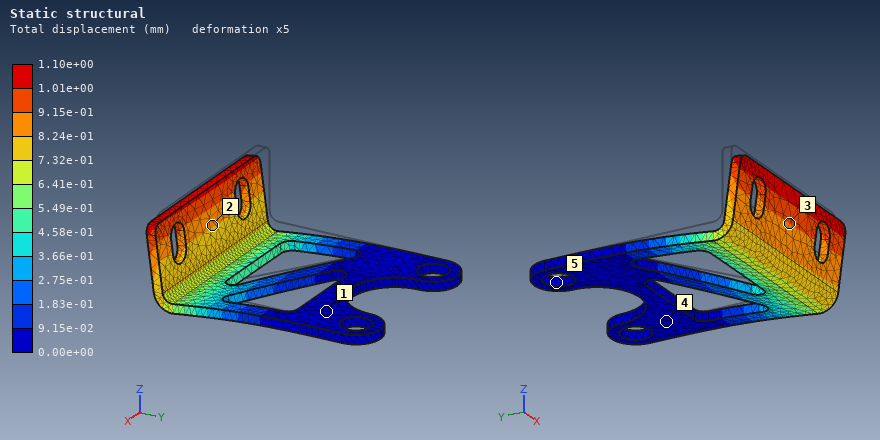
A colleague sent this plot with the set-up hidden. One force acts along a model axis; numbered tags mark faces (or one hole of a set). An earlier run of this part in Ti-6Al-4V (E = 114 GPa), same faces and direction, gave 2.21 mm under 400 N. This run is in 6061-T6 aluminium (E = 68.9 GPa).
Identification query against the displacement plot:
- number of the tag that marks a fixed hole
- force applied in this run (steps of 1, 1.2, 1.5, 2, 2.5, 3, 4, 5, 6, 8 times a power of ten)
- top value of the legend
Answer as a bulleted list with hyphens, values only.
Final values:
- 5
- 120 N
- 1.10e+00 mm
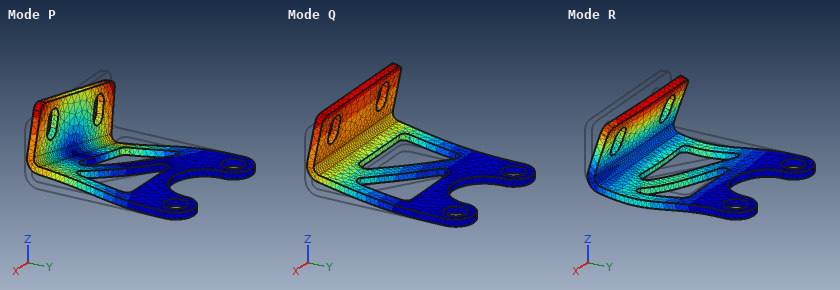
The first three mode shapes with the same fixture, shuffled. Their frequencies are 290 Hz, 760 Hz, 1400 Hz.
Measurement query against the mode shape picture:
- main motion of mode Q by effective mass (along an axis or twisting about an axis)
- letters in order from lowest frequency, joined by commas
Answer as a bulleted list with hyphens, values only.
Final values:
- along Z
- Q, P, R
